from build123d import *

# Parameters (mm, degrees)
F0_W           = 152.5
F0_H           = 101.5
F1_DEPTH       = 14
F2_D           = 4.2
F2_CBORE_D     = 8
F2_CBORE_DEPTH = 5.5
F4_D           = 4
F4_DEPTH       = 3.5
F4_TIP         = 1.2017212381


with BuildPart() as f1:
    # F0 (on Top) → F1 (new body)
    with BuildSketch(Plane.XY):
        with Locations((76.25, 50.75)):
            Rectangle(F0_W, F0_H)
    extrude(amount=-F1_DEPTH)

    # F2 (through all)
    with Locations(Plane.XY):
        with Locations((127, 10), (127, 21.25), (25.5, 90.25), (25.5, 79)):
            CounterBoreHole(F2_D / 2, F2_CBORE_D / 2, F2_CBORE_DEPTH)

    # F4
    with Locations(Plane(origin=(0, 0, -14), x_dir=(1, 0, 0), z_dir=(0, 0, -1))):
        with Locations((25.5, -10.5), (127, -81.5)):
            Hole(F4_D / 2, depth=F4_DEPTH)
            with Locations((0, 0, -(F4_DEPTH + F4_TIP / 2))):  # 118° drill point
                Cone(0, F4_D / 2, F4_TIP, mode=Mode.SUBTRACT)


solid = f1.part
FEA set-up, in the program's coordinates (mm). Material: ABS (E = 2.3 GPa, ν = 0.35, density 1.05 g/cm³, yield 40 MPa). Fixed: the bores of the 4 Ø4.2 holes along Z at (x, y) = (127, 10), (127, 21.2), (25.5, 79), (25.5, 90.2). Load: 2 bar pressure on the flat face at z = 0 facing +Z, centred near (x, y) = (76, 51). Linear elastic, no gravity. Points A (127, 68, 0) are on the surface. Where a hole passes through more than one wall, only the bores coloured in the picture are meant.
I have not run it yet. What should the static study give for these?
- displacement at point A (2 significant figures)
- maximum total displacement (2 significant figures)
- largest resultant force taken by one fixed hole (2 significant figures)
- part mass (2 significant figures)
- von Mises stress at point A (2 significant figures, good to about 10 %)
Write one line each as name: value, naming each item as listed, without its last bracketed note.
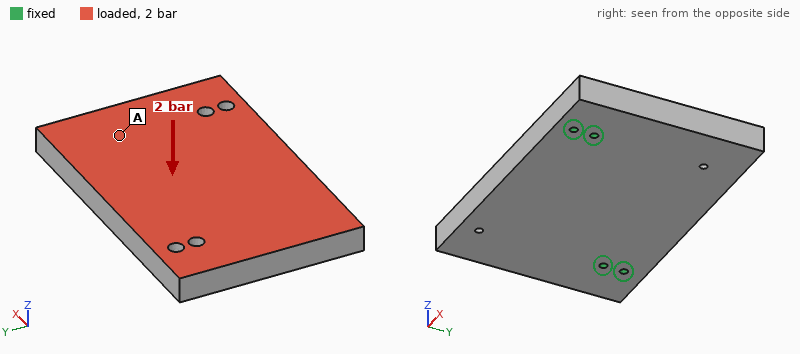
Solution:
displacement at point A: 0.91 mm
maximum total displacement: 1.7 mm
largest resultant force taken by one fixed hole: 1.8 kN
part mass: 230 g
von Mises stress at point A: 4.7 MPa
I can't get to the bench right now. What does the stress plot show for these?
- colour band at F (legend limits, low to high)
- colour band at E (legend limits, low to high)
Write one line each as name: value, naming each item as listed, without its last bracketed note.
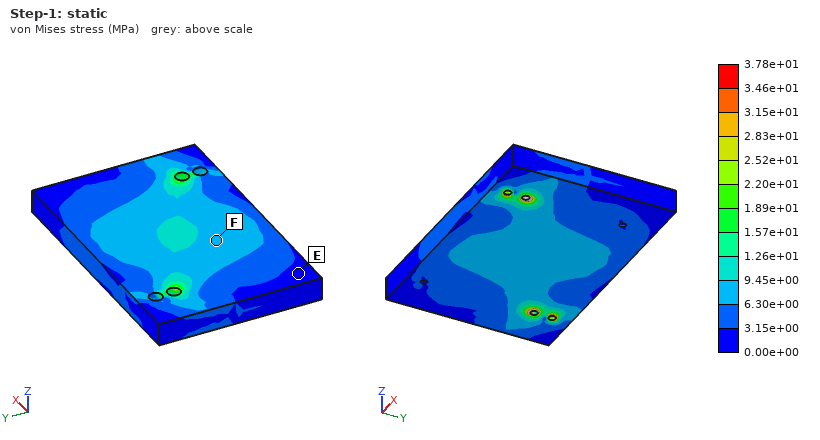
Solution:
colour band at F: 6.30e+00 to 9.45e+00 MPa
colour band at E: 0.00e+00 to 3.15e+00 MPa
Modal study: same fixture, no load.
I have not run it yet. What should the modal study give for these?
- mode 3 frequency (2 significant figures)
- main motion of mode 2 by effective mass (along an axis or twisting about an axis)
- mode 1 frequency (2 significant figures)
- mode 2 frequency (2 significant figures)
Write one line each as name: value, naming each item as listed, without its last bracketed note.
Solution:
mode 3 frequency: 1100 Hz
main motion of mode 2 by effective mass: along Z
mode 1 frequency: 430 Hz
mode 2 frequency: 620 Hz
